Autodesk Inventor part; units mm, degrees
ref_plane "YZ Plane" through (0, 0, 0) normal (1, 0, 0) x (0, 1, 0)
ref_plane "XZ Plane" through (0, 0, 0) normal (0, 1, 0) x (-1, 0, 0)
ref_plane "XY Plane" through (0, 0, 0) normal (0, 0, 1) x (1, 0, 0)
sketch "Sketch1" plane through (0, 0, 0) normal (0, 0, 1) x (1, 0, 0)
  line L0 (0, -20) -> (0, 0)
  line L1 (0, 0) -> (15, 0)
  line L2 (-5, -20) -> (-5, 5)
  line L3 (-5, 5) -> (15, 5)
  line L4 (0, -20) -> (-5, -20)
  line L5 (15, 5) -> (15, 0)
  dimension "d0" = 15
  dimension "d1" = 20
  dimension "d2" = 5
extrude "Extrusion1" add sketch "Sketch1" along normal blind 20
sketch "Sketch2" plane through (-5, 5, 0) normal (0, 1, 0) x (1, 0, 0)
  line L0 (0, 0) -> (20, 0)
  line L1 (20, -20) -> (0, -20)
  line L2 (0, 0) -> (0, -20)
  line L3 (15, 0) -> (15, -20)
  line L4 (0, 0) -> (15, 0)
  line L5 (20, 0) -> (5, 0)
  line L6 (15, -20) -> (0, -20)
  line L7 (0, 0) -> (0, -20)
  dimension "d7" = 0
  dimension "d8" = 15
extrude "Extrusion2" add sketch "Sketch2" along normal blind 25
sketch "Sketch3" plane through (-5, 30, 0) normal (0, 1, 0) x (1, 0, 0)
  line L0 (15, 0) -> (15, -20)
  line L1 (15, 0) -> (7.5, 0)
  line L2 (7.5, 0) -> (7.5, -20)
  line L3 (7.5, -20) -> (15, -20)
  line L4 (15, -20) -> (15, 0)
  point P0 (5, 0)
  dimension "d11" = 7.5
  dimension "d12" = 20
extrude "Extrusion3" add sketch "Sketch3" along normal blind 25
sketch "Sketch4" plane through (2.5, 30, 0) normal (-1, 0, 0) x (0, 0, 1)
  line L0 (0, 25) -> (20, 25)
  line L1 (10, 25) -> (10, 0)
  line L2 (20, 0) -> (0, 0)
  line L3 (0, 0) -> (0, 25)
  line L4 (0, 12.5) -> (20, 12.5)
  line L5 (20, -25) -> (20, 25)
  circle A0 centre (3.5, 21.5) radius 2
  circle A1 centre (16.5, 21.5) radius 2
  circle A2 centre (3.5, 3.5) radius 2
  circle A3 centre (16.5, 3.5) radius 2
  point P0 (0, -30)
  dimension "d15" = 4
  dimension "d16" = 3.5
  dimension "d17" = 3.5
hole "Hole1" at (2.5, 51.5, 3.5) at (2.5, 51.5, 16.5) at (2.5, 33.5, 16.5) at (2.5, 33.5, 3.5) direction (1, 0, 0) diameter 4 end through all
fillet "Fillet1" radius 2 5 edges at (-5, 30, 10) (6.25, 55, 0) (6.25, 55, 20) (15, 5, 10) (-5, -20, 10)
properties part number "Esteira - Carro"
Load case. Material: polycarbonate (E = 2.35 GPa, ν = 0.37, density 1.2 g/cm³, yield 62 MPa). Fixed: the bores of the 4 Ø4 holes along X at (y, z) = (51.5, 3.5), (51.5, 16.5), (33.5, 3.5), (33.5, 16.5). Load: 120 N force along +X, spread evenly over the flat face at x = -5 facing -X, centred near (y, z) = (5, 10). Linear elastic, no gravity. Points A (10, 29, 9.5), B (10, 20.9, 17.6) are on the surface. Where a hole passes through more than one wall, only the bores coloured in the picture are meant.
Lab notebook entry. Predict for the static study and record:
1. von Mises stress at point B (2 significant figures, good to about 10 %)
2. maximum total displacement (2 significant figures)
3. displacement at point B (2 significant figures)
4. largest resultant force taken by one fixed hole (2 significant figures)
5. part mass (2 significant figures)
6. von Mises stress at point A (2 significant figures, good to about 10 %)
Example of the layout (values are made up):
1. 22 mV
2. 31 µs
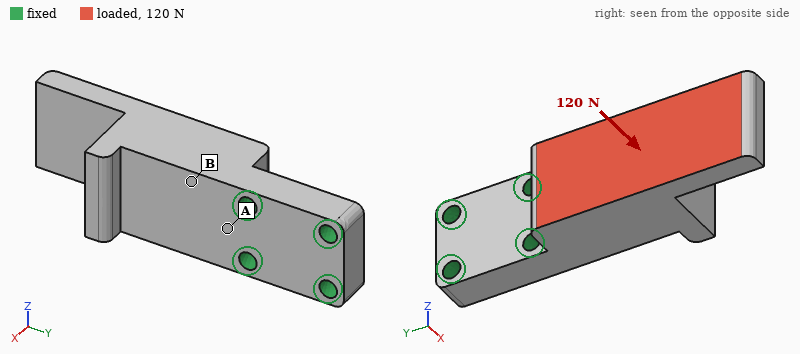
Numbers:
1. 3.6 MPa
2. 0.80 mm
3. 0.12 mm
4. 71 N
5. 18 g
6. 8.9 MPa
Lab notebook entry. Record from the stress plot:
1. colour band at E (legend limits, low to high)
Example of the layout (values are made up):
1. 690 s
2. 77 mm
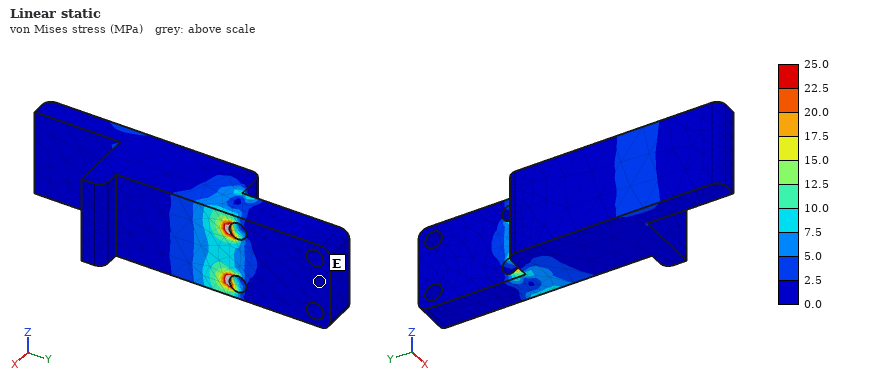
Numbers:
1. 0.0 to 2.5 MPa
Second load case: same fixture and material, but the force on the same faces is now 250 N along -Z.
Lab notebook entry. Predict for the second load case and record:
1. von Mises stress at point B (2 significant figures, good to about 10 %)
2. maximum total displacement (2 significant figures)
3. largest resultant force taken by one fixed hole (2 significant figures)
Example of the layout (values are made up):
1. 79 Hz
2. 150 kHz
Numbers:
1. 3.7 MPa
2. 0.40 mm
3. 520 N
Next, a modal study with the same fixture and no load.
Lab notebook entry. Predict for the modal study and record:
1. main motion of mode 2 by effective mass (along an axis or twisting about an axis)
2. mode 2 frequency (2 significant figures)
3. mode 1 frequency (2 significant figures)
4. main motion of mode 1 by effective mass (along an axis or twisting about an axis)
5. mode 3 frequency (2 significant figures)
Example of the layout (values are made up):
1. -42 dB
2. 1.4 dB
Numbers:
1. along Z
2. 1700 Hz
3. 830 Hz
4. along X
5. 2800 Hz
